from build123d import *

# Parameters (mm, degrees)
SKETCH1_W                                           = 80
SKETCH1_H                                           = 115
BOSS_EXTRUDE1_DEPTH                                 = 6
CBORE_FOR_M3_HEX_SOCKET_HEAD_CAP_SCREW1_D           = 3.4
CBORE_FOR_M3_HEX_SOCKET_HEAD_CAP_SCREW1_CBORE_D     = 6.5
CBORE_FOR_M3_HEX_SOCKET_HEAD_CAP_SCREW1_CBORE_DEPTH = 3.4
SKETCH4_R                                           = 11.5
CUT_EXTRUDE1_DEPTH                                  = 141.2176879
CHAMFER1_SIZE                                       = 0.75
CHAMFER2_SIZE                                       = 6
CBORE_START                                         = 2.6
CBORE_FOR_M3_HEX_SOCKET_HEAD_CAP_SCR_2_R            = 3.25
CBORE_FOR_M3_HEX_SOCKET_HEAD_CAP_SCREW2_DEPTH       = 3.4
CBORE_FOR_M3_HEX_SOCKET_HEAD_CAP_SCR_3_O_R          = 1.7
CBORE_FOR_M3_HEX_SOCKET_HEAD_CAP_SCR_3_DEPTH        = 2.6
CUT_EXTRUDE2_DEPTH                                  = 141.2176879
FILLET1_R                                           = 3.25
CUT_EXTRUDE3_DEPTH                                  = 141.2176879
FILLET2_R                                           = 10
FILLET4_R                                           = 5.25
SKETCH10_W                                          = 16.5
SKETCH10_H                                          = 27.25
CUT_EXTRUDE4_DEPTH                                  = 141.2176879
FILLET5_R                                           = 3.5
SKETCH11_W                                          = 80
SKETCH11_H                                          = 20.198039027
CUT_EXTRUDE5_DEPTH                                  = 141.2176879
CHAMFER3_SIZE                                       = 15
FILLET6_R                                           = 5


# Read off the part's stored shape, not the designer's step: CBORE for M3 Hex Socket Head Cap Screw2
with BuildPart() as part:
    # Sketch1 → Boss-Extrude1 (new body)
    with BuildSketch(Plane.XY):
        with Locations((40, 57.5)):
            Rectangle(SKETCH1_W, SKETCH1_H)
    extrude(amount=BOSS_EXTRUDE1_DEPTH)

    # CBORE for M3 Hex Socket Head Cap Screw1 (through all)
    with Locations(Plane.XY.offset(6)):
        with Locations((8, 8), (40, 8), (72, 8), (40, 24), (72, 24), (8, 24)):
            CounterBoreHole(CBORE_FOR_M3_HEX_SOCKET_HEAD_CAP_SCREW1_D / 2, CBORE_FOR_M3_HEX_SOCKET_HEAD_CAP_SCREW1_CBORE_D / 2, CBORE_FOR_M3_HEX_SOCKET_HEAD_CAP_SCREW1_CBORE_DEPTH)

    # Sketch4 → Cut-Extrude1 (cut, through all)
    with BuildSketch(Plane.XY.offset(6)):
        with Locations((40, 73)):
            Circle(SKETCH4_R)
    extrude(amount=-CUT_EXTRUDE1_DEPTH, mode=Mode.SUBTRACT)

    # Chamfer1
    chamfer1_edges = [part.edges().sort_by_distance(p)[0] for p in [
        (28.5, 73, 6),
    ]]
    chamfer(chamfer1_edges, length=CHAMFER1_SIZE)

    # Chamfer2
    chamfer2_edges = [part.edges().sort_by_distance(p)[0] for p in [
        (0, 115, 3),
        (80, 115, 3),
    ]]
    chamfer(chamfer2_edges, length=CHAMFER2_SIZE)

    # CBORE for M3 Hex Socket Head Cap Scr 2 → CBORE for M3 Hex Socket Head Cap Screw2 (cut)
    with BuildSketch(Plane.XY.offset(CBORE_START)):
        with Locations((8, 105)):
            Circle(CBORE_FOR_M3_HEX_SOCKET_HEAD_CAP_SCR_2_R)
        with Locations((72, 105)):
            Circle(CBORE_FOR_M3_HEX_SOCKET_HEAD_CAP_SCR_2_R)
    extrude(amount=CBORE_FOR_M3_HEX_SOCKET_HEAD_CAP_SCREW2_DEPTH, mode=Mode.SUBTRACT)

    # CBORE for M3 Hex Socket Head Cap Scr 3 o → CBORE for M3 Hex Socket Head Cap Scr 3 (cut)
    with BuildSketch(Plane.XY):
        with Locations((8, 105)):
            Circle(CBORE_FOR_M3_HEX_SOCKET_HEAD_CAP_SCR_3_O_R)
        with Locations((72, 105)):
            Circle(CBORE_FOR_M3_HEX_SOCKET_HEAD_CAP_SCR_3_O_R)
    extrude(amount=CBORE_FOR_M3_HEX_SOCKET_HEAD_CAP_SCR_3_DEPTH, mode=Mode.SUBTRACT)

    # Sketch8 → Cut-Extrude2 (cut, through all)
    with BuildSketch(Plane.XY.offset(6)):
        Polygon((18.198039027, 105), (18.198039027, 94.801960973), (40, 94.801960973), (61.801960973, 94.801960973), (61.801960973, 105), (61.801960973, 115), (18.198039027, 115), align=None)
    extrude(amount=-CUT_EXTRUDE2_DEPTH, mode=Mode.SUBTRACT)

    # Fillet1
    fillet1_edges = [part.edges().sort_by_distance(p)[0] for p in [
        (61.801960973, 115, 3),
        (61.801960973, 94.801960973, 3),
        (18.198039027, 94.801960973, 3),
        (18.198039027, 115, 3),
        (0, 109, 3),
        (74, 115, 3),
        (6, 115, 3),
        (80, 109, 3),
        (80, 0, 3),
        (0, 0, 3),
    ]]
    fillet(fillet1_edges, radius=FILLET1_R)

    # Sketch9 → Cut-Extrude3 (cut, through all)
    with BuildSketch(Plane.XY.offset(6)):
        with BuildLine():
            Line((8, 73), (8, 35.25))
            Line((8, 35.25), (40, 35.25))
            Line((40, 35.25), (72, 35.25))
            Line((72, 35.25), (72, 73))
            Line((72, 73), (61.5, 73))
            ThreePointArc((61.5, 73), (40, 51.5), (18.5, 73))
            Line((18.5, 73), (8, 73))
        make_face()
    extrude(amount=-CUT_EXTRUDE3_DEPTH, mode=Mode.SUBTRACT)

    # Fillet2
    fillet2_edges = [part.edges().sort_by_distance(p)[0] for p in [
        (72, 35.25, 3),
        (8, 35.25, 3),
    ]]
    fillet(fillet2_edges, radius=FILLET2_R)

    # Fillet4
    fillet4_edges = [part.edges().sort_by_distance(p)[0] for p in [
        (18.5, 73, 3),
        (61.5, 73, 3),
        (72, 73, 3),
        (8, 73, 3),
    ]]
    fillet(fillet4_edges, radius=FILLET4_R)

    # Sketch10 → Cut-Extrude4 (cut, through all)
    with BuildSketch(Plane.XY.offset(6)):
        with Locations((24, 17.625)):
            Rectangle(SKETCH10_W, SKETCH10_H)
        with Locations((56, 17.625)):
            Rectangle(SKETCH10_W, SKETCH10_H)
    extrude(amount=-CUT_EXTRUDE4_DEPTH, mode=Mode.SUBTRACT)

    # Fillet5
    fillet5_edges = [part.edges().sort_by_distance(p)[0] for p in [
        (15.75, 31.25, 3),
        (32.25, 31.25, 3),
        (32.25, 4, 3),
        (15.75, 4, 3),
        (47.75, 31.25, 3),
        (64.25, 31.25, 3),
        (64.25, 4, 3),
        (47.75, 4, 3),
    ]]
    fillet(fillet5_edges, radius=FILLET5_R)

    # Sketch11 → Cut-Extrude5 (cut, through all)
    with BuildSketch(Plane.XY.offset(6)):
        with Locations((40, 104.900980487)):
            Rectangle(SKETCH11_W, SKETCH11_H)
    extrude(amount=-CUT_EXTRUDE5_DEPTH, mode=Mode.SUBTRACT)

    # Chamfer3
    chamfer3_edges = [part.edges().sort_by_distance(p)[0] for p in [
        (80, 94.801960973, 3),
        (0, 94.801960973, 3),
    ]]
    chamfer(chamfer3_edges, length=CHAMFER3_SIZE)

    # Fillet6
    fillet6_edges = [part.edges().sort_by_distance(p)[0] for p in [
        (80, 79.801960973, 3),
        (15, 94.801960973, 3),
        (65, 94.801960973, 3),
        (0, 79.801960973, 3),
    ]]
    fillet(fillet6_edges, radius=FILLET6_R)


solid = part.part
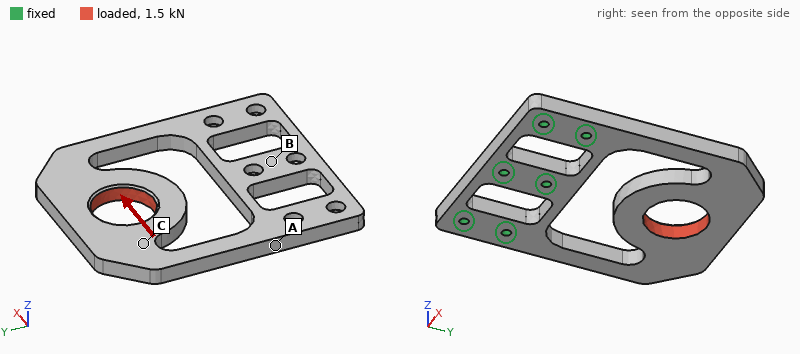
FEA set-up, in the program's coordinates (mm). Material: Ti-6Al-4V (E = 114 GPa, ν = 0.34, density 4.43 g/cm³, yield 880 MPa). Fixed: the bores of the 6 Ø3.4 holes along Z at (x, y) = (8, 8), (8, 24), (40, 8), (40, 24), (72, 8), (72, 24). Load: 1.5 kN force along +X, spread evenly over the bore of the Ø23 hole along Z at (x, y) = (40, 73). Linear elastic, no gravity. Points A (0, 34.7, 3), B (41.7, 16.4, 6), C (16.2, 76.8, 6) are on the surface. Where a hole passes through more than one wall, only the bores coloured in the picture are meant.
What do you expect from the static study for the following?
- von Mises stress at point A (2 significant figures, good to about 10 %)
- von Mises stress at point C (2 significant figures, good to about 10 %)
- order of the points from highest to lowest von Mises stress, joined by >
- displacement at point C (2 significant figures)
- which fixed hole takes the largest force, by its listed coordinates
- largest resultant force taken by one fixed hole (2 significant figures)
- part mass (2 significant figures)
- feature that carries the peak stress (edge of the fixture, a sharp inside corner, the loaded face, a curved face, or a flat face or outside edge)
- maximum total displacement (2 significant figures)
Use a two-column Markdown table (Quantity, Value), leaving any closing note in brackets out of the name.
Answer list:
| Quantity | Value |
|---|---|
| von Mises stress at point A | 110 MPa |
| von Mises stress at point C | 33 MPa |
| order of the points from highest to lowest von Mises stress, joined by > | A > C > B |
| displacement at point C | 0.19 mm |
| which fixed hole takes the largest force, by its listed coordinates | (40, 24) |
| largest resultant force taken by one fixed hole | 1.4 kN |
| part mass | 110 g |
| feature that carries the peak stress | a curved face |
| maximum total displacement | 0.20 mm |
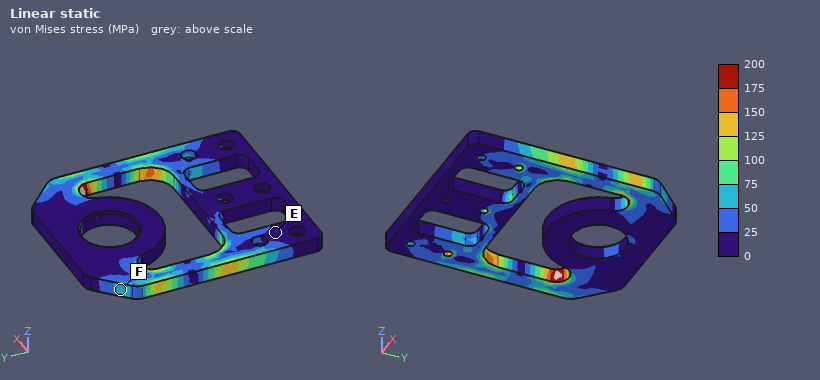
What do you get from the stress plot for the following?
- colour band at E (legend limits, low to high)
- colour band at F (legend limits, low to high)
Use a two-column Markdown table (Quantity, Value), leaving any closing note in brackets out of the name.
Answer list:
| Quantity | Value |
|---|---|
| colour band at E | 0 to 25 MPa |
| colour band at F | 50 to 75 MPa |
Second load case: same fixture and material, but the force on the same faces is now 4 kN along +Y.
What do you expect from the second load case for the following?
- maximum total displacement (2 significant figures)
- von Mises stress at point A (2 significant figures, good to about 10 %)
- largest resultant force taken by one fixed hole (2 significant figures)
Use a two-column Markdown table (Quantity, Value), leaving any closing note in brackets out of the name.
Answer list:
| Quantity | Value |
|---|---|
| maximum total displacement | 92 µm |
| von Mises stress at point A | 60 MPa |
| largest resultant force taken by one fixed hole | 1.5 kN |
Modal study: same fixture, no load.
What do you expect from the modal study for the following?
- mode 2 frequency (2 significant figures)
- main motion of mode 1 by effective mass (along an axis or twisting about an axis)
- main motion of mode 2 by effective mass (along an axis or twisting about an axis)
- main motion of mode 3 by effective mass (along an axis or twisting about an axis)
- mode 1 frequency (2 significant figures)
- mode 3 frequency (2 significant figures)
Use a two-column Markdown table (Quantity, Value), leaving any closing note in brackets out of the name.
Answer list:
| Quantity | Value |
|---|---|
| mode 2 frequency | 1600 Hz |
| main motion of mode 1 by effective mass | along Z |
| main motion of mode 2 by effective mass | twisting about Y |
| main motion of mode 3 by effective mass | along X |
| mode 1 frequency | 560 Hz |
| mode 3 frequency | 1900 Hz |
